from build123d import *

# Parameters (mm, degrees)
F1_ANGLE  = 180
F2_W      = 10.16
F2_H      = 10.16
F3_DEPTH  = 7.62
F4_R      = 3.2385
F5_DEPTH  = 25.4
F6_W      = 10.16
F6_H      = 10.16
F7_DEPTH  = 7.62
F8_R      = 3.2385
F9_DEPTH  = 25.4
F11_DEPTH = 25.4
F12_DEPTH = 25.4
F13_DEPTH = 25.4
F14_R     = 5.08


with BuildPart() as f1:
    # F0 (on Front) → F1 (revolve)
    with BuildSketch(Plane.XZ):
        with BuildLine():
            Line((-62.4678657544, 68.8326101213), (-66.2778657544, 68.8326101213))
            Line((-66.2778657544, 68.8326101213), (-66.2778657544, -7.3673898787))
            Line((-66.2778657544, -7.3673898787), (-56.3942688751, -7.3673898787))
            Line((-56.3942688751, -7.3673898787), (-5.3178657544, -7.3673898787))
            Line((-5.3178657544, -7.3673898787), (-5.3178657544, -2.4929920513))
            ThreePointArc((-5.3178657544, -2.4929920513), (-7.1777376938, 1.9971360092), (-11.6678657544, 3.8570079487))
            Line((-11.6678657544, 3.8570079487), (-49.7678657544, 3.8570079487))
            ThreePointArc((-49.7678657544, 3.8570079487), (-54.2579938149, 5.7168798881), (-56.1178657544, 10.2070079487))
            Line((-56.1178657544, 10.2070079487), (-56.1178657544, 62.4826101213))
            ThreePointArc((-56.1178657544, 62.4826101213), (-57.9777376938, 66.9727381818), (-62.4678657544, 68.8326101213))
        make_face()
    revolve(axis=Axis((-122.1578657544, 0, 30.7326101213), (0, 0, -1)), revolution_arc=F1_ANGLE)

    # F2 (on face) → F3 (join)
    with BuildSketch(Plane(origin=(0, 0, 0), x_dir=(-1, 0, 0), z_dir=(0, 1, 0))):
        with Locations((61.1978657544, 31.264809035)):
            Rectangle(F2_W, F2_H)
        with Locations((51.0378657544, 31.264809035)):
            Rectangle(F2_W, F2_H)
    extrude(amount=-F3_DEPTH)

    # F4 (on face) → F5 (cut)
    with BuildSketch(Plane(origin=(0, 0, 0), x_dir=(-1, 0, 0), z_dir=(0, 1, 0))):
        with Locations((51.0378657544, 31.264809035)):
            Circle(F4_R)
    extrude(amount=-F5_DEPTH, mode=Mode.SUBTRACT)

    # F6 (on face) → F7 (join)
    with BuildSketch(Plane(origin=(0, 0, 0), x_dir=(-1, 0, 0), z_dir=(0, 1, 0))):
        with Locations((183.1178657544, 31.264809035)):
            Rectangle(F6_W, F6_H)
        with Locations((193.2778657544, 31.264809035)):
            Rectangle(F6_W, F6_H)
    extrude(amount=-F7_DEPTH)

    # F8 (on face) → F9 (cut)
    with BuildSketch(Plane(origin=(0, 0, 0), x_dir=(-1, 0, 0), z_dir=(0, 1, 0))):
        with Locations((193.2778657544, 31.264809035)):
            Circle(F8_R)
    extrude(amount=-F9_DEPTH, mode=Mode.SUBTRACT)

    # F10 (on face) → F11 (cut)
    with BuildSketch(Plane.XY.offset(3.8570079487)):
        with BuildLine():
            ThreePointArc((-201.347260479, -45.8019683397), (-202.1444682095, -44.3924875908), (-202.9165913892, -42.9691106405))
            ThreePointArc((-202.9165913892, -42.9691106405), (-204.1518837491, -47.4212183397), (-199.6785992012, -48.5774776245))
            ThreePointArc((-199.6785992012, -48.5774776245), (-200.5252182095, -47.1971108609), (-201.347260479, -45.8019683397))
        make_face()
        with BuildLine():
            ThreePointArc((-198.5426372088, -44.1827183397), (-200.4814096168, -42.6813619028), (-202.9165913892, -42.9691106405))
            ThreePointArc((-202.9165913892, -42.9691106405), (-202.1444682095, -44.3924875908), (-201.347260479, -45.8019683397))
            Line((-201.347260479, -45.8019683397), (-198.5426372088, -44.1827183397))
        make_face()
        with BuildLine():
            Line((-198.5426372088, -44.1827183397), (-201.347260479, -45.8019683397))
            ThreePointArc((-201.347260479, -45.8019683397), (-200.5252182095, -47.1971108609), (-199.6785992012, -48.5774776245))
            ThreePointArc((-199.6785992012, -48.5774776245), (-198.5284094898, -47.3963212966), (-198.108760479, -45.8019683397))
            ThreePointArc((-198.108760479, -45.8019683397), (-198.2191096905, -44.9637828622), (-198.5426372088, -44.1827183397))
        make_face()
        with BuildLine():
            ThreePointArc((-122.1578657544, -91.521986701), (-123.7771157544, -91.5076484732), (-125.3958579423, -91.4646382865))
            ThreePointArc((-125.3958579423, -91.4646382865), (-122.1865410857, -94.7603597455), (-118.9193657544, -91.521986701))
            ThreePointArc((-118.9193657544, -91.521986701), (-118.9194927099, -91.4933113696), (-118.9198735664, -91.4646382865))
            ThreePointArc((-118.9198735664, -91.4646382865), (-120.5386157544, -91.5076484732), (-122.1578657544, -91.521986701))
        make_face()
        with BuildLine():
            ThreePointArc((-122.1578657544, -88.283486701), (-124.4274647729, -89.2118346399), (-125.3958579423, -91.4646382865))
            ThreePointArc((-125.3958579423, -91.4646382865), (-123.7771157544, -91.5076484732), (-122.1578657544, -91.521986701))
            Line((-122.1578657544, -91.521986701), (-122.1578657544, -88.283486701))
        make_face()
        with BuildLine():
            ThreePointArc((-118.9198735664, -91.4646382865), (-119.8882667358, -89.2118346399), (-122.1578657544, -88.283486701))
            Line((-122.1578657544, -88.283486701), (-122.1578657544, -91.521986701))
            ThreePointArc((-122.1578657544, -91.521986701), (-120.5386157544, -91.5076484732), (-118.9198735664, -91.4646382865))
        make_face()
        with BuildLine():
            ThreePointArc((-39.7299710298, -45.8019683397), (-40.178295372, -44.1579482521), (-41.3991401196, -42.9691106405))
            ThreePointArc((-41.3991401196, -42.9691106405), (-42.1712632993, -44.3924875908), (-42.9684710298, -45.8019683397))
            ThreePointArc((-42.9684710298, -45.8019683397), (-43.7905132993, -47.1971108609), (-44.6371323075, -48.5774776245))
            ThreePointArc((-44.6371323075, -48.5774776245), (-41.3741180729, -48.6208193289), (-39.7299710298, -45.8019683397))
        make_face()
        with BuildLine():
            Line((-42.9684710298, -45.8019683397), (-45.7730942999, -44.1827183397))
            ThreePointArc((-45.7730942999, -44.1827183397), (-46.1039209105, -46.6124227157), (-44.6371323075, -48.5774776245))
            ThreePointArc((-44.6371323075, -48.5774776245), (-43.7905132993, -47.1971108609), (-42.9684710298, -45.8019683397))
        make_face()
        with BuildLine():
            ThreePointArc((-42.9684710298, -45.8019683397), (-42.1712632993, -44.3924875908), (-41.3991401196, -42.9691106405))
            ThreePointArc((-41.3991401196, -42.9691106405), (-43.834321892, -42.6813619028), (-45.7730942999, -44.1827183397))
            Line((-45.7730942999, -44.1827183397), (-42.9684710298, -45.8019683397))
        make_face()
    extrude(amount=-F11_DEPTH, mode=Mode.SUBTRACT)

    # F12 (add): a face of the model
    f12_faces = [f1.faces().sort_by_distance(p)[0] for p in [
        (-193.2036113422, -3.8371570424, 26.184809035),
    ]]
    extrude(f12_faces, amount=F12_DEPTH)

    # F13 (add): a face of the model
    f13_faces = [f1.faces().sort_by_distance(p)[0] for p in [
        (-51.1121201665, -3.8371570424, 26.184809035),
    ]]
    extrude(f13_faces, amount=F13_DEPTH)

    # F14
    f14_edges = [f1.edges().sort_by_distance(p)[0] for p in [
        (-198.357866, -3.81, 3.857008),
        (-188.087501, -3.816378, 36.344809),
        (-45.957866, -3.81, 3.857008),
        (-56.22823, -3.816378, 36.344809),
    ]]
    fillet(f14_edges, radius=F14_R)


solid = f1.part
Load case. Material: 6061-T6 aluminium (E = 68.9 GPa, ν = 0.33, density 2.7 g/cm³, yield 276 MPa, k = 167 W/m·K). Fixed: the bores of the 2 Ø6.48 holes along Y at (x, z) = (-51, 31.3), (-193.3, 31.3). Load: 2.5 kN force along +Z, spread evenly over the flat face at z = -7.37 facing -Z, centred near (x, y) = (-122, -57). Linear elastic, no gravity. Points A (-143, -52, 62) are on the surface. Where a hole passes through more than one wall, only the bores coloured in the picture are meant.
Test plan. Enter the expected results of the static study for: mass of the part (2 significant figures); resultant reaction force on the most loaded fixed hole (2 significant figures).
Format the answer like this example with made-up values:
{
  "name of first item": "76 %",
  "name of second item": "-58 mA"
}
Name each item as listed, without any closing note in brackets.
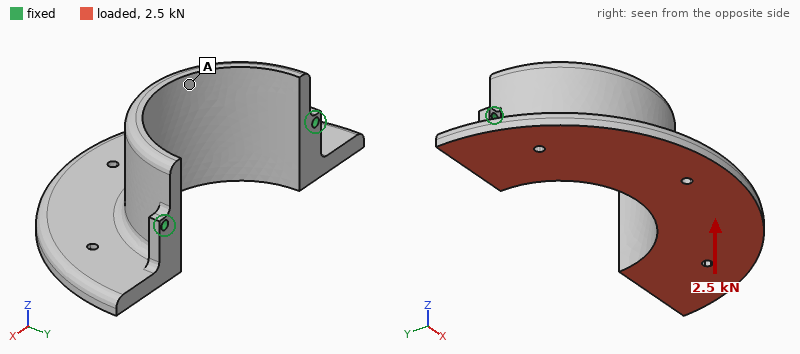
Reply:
{
  "mass of the part": "840 g",
  "resultant reaction force on the most loaded fixed hole": "1.3 kN"
}
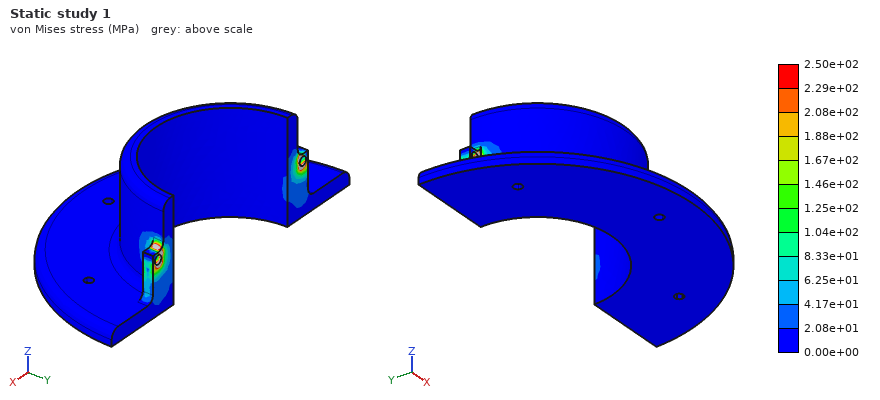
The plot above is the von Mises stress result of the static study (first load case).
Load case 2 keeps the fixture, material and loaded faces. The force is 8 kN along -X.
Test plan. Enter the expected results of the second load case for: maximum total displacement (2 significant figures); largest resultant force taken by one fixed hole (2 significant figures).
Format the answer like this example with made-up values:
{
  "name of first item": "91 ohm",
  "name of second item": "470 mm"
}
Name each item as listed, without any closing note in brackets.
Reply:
{
  "maximum total displacement": "0.16 mm",
  "largest resultant force taken by one fixed hole": "5.4 kN"
}
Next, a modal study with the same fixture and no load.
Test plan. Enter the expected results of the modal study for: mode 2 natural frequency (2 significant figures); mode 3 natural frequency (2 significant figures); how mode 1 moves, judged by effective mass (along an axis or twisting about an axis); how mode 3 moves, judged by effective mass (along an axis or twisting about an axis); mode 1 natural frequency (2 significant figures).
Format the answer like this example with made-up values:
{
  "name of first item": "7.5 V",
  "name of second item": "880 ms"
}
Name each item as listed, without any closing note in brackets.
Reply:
{
  "mode 2 natural frequency": "1200 Hz",
  "mode 3 natural frequency": "2100 Hz",
  "how mode 1 moves, judged by effective mass": "along Z",
  "how mode 3 moves, judged by effective mass": "along X",
  "mode 1 natural frequency": "410 Hz"
}
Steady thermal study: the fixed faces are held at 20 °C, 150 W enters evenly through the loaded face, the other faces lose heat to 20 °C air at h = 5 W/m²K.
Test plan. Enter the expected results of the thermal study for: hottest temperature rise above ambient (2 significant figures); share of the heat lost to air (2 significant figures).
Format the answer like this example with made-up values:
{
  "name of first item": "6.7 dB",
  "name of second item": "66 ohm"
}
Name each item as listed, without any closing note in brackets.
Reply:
{
  "hottest temperature rise above ambient": "56 K",
  "share of the heat lost to air": "6.7 %"
}
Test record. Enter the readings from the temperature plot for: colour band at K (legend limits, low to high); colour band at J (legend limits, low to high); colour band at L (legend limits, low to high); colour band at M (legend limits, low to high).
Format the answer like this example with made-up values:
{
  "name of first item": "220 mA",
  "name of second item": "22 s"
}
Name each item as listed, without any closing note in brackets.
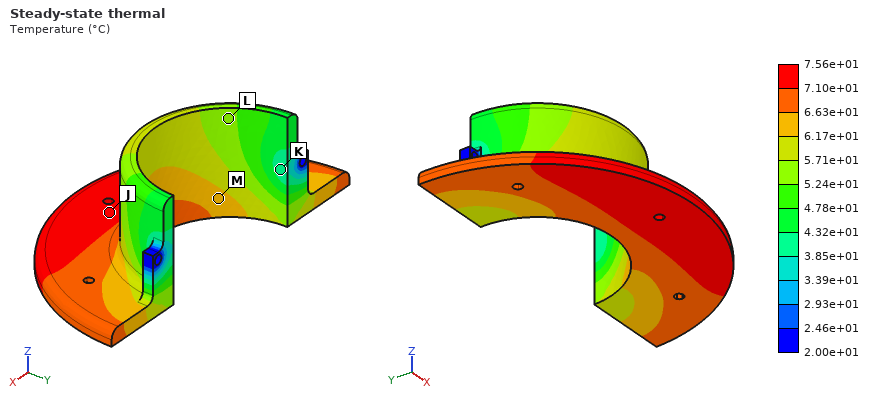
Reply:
{
  "colour band at K": "3.85e+01 to 4.32e+01 °C",
  "colour band at J": "7.10e+01 to 7.56e+01 °C",
  "colour band at L": "5.24e+01 to 5.71e+01 °C",
  "colour band at M": "6.17e+01 to 6.63e+01 °C"
}
